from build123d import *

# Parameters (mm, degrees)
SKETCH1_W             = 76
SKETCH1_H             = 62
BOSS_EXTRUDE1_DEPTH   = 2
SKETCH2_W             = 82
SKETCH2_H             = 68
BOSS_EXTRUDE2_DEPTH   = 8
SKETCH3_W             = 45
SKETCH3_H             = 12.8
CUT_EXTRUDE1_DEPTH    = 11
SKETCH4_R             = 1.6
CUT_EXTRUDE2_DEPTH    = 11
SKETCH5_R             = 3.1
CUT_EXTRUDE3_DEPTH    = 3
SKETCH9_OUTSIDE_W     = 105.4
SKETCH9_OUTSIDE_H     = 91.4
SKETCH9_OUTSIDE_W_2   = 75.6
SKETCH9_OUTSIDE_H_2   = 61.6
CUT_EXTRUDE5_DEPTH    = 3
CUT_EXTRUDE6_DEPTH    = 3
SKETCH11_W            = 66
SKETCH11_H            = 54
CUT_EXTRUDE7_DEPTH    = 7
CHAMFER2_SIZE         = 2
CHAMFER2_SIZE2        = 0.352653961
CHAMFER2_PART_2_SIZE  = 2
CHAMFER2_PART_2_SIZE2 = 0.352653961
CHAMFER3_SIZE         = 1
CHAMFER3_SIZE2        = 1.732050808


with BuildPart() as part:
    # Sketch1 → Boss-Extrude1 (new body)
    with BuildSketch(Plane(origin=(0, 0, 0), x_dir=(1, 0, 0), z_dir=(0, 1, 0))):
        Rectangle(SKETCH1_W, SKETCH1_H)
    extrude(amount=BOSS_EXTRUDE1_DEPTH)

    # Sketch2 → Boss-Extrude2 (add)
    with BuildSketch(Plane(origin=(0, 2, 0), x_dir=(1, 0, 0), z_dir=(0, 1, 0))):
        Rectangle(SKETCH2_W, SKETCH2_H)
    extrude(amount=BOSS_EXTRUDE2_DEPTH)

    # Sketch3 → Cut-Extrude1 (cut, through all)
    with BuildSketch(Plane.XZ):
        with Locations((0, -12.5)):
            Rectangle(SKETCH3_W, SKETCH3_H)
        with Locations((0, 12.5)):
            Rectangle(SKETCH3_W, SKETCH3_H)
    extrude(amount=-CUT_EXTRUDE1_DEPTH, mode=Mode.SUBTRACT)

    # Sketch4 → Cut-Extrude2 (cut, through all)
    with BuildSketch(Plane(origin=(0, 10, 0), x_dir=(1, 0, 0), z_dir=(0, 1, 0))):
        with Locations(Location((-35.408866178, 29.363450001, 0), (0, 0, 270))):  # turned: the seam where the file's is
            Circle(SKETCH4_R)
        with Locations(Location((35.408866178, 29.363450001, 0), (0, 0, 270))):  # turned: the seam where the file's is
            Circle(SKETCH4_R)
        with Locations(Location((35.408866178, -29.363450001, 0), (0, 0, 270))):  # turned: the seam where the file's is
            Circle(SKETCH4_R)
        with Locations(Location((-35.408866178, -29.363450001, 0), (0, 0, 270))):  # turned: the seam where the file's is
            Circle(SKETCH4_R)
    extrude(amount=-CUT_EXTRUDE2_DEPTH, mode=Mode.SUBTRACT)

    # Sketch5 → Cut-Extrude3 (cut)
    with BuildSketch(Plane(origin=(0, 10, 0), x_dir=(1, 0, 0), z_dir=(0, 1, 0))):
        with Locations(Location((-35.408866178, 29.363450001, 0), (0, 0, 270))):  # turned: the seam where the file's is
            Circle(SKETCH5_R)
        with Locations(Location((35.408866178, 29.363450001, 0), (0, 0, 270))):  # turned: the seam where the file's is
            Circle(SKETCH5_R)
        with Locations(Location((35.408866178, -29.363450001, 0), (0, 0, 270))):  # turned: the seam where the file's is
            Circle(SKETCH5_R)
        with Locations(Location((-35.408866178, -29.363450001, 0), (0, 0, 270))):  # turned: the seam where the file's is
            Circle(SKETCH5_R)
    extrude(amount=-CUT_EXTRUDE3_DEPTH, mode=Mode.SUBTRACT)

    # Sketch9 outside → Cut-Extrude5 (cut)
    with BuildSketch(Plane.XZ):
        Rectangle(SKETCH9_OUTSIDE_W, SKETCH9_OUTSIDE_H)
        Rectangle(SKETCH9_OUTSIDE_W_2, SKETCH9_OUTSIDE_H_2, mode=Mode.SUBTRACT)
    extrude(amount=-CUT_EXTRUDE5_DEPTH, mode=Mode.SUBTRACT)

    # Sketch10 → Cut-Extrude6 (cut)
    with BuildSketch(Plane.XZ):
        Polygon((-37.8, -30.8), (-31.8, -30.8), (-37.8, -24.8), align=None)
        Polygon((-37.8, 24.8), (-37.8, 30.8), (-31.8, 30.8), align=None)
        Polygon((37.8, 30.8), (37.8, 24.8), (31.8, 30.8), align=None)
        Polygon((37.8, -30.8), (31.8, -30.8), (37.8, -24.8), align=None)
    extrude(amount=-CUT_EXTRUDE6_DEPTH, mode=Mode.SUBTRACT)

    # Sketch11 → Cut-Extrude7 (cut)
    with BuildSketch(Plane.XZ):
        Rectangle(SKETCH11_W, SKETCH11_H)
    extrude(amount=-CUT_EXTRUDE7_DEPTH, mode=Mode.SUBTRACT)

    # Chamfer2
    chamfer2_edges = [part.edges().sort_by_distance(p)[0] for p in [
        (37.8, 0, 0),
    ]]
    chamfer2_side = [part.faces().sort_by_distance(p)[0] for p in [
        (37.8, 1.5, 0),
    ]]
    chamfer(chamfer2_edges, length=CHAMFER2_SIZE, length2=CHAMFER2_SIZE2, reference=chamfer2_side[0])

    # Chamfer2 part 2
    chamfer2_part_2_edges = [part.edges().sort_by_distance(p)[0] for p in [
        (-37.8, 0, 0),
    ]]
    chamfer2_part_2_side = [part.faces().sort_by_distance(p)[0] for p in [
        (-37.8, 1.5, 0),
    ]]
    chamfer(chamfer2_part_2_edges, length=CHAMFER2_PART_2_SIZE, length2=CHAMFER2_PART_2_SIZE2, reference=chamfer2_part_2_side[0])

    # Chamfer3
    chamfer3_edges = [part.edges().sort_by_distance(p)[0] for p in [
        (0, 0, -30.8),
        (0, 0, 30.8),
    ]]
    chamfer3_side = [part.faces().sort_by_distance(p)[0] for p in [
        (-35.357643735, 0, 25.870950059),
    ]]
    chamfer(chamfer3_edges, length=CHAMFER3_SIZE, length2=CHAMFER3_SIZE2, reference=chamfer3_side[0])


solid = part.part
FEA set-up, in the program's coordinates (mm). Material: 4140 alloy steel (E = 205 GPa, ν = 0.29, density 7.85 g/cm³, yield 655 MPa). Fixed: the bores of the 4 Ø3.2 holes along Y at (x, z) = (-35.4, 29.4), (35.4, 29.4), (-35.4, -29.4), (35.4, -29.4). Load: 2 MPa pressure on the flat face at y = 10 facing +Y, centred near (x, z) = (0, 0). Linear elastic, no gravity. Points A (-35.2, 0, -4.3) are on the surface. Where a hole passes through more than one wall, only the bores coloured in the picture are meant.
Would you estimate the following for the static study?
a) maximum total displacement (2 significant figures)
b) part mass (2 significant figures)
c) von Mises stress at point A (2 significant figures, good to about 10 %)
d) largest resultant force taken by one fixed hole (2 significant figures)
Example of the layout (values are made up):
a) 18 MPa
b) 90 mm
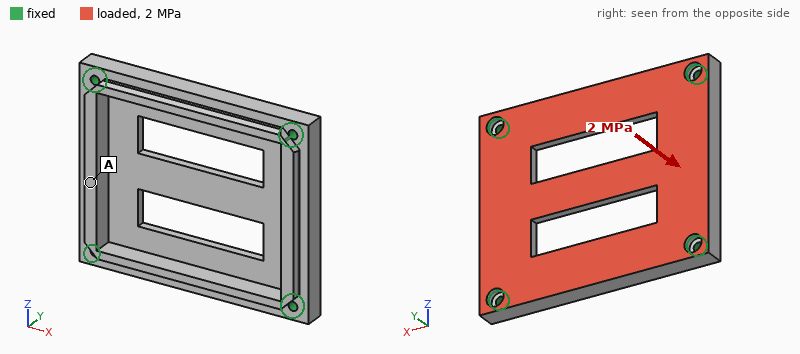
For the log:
a) 0.24 mm
b) 190 g
c) 84 MPa
d) 2.7 kN
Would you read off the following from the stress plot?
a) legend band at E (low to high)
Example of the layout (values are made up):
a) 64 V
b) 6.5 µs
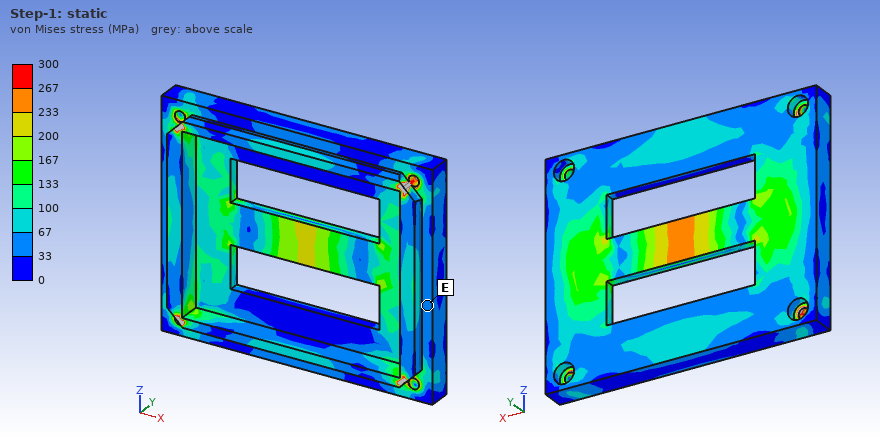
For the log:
a) 33 to 67 MPa
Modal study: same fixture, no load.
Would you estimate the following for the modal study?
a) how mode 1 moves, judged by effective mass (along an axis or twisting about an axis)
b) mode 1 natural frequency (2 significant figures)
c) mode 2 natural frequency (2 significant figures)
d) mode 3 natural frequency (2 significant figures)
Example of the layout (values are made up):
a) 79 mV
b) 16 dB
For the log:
a) along Y
b) 3800 Hz
c) 6900 Hz
d) 6900 Hz
